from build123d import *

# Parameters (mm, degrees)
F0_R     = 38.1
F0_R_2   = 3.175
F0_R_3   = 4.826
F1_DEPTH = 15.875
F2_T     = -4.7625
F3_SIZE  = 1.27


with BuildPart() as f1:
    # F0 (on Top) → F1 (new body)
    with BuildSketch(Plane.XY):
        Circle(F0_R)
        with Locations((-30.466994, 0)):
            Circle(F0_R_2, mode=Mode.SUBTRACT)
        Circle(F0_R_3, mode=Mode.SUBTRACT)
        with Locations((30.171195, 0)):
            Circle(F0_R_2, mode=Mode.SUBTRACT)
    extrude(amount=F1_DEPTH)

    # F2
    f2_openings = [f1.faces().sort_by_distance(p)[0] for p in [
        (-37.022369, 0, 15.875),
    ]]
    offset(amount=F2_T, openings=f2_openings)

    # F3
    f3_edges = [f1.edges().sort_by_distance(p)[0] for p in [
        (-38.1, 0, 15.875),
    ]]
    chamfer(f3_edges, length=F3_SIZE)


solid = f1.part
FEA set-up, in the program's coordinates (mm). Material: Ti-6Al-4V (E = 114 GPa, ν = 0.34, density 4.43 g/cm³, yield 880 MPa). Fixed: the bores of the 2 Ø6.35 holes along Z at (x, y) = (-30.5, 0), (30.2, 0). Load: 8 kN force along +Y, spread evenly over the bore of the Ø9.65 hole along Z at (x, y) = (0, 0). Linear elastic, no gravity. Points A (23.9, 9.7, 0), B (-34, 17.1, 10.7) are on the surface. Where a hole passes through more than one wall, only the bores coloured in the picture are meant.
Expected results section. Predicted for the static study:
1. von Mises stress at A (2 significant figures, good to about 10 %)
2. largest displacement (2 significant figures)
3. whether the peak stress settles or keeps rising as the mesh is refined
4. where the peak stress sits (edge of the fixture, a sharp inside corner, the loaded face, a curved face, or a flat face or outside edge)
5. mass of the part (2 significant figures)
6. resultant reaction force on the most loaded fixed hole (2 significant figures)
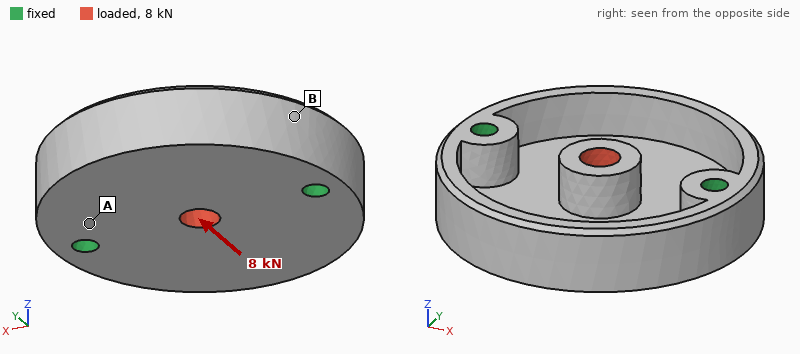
29 MPa
63 µm
keeps rising
a sharp inside corner
170 g
4.0 kN
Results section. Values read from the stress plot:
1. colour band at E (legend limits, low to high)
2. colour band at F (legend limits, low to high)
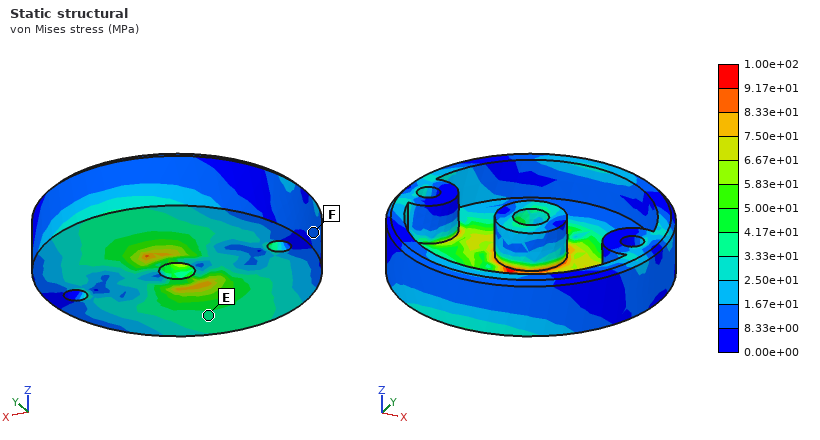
3.33e+01 to 4.17e+01 MPa
8.33e+00 to 1.67e+01 MPa
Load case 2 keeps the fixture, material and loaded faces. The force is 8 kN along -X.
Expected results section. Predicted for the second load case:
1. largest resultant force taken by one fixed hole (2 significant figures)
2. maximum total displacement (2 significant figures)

4.1 kN
42 µm
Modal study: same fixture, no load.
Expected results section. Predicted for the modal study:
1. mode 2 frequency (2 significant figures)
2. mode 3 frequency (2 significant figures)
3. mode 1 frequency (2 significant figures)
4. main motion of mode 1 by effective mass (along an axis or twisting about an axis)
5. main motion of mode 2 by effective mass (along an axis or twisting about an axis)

5500 Hz
9800 Hz
4900 Hz
twisting about X
along Z
